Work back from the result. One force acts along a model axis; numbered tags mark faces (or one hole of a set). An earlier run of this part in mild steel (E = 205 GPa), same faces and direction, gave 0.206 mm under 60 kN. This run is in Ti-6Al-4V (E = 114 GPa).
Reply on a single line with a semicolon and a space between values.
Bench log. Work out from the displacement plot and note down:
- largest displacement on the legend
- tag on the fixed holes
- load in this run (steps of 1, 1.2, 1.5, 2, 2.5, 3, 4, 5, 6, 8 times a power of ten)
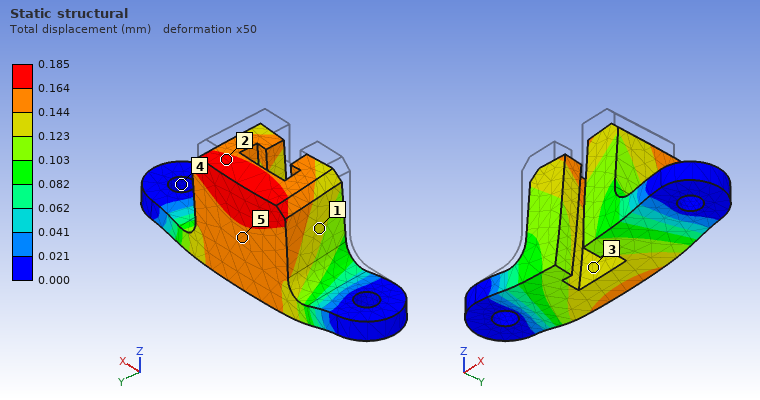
0.185 mm; 4; 30 kN
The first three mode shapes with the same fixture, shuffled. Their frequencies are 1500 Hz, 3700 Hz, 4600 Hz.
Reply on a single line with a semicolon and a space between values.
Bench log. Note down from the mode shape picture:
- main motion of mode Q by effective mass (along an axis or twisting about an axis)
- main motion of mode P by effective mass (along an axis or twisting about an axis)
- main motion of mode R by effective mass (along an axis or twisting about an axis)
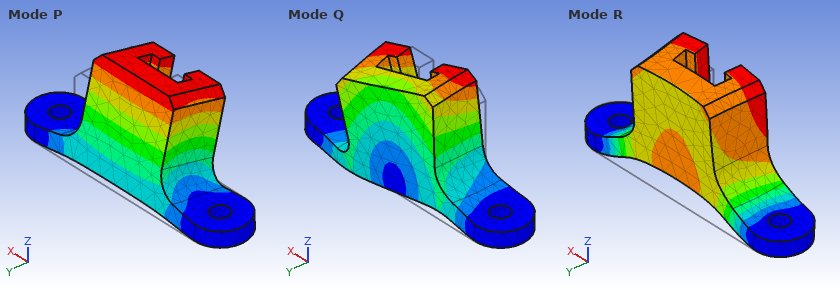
along X; along Y; along Z
